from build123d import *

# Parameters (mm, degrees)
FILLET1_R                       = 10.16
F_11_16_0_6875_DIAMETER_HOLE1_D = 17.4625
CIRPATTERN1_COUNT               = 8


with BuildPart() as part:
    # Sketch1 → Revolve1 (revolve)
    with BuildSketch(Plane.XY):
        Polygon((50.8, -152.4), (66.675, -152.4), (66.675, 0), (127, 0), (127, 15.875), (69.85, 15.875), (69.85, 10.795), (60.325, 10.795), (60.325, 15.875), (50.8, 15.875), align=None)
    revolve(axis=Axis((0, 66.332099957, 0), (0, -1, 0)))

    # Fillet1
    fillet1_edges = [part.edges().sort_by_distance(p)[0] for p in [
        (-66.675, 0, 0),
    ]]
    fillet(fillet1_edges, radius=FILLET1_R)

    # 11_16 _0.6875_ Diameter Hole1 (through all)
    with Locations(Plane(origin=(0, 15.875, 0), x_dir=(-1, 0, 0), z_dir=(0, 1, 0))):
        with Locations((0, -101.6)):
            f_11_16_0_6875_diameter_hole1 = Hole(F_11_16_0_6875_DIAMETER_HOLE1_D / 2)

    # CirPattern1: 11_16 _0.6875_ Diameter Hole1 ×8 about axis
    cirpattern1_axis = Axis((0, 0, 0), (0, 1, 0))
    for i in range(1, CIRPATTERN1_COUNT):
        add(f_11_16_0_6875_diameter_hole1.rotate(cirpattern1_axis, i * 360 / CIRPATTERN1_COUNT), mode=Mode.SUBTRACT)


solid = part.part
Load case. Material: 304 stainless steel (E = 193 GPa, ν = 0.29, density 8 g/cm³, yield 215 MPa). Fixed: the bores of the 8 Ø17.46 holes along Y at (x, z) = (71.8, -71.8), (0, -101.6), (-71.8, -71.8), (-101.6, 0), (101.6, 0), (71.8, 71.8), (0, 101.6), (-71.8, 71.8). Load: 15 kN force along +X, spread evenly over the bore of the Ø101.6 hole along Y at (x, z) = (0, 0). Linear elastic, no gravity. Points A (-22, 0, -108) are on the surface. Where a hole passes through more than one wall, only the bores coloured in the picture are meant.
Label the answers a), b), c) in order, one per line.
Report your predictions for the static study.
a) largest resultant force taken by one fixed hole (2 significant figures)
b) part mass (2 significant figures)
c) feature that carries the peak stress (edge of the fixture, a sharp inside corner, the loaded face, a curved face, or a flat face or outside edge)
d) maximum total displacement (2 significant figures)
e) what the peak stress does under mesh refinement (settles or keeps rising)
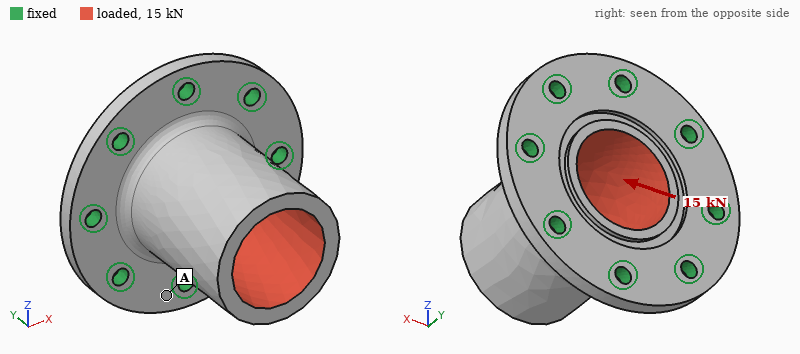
a) 4.7 kN
b) 12 kg
c) edge of the fixture
d) 22 µm
e) keeps rising
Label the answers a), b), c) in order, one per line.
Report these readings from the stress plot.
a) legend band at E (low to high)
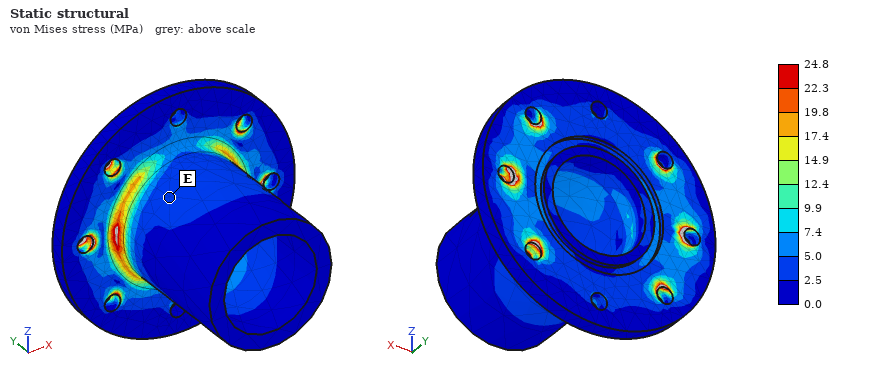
a) 2.5 to 5.0 MPa
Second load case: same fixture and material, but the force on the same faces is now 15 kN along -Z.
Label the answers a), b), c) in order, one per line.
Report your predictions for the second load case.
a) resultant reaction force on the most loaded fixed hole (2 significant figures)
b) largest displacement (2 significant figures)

a) 4.7 kN
b) 22 µm
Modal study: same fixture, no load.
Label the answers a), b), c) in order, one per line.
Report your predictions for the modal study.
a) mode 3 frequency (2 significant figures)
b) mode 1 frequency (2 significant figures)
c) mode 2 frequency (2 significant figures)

a) 3100 Hz
b) 1700 Hz
c) 1700 Hz
